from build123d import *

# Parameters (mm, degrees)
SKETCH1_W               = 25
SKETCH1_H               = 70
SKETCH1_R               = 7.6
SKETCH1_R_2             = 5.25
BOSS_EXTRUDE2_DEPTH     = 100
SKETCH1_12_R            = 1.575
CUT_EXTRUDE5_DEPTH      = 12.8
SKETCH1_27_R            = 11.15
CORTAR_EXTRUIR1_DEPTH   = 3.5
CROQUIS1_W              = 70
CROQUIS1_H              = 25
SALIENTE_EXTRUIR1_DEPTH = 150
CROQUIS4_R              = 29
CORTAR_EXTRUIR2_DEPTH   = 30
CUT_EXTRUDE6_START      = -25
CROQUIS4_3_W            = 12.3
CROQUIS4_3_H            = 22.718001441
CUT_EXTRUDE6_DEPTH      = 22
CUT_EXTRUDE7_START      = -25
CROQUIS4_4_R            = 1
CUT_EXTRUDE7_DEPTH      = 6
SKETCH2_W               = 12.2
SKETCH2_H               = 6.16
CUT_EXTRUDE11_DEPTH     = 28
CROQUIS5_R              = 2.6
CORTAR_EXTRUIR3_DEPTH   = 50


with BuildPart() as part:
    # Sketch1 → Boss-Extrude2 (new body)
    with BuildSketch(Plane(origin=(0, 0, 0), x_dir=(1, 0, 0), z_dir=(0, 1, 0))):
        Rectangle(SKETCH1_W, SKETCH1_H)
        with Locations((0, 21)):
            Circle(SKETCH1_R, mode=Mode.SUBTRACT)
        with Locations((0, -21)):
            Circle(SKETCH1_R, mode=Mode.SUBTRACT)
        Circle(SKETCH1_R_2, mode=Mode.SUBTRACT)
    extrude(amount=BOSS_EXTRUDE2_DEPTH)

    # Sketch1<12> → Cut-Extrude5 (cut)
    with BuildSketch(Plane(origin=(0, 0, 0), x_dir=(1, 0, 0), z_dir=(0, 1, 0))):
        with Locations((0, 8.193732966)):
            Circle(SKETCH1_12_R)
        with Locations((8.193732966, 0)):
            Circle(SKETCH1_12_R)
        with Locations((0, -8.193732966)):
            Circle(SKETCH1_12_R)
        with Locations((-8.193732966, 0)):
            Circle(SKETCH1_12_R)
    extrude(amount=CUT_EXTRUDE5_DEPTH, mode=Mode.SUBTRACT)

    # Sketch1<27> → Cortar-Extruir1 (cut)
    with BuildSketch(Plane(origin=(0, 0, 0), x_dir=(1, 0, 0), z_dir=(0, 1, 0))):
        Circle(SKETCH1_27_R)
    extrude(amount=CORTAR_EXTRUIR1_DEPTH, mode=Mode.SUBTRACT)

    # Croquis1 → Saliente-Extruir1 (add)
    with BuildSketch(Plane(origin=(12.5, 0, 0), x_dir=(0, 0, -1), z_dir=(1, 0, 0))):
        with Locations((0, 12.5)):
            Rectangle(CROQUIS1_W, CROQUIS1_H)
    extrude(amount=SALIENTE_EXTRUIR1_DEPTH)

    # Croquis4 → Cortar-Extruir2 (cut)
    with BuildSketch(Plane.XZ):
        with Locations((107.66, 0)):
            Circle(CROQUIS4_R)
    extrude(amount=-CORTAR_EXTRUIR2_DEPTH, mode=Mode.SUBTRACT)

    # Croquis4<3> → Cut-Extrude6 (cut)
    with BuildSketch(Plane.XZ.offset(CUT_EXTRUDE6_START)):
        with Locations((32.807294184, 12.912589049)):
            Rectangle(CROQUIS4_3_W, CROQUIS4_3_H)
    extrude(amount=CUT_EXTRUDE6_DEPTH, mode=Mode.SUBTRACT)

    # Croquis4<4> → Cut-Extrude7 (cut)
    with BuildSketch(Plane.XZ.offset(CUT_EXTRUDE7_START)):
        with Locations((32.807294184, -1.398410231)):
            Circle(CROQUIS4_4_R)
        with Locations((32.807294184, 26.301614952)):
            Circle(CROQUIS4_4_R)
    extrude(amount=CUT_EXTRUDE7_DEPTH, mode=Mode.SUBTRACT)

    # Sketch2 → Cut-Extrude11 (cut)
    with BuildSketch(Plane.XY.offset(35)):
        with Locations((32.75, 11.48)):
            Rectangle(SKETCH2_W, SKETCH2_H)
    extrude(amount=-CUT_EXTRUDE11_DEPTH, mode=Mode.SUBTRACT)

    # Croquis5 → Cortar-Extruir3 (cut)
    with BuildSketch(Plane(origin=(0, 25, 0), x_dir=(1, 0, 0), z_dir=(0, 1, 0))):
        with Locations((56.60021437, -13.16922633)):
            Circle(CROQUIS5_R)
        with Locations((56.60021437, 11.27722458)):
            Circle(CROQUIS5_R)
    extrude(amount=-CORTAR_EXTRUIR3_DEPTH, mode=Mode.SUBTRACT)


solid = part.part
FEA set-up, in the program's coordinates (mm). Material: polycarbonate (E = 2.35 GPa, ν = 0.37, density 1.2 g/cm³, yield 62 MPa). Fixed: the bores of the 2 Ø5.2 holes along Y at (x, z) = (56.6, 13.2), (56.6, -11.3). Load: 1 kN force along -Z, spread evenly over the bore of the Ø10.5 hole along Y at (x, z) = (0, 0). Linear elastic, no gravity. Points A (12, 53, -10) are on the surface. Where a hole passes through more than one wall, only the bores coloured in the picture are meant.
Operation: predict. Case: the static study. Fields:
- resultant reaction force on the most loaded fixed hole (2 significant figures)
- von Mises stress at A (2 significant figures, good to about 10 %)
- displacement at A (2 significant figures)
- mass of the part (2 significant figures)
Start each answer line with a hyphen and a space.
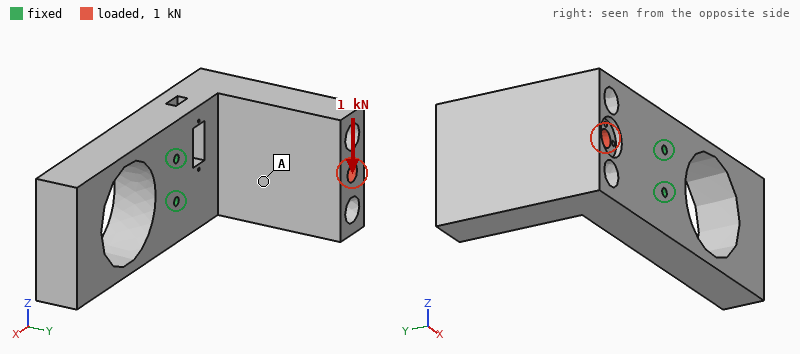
- 2.2 kN
- 1.6 MPa
- 0.59 mm
- 380 g
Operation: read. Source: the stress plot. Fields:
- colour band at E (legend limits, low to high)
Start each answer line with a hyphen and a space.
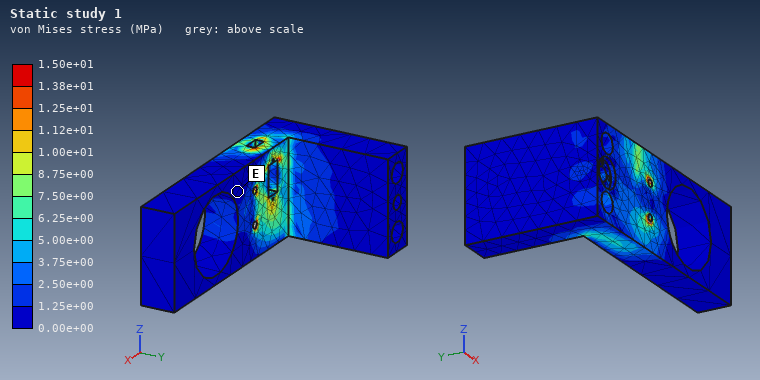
- 0.00e+00 to 1.25e+00 MPa
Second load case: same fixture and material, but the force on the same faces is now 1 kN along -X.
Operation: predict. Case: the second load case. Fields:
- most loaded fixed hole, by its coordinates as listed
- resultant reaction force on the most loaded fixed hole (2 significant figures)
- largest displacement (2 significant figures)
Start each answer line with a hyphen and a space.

- (56.6, -11.3)
- 570 N
- 1.8 mm
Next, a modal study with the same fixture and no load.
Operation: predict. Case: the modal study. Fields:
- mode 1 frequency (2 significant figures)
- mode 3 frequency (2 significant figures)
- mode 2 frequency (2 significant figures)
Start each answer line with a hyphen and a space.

- 310 Hz
- 420 Hz
- 350 Hz
